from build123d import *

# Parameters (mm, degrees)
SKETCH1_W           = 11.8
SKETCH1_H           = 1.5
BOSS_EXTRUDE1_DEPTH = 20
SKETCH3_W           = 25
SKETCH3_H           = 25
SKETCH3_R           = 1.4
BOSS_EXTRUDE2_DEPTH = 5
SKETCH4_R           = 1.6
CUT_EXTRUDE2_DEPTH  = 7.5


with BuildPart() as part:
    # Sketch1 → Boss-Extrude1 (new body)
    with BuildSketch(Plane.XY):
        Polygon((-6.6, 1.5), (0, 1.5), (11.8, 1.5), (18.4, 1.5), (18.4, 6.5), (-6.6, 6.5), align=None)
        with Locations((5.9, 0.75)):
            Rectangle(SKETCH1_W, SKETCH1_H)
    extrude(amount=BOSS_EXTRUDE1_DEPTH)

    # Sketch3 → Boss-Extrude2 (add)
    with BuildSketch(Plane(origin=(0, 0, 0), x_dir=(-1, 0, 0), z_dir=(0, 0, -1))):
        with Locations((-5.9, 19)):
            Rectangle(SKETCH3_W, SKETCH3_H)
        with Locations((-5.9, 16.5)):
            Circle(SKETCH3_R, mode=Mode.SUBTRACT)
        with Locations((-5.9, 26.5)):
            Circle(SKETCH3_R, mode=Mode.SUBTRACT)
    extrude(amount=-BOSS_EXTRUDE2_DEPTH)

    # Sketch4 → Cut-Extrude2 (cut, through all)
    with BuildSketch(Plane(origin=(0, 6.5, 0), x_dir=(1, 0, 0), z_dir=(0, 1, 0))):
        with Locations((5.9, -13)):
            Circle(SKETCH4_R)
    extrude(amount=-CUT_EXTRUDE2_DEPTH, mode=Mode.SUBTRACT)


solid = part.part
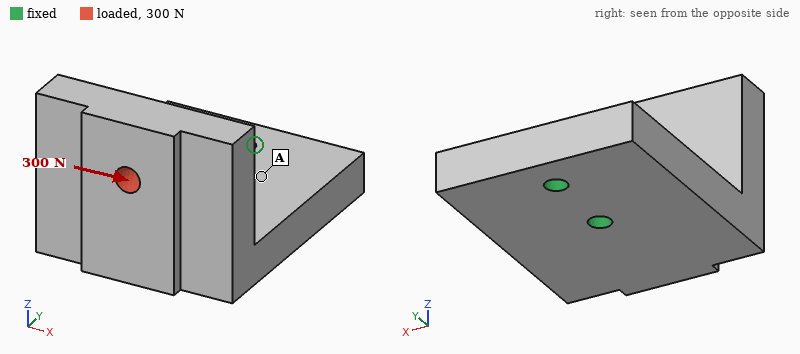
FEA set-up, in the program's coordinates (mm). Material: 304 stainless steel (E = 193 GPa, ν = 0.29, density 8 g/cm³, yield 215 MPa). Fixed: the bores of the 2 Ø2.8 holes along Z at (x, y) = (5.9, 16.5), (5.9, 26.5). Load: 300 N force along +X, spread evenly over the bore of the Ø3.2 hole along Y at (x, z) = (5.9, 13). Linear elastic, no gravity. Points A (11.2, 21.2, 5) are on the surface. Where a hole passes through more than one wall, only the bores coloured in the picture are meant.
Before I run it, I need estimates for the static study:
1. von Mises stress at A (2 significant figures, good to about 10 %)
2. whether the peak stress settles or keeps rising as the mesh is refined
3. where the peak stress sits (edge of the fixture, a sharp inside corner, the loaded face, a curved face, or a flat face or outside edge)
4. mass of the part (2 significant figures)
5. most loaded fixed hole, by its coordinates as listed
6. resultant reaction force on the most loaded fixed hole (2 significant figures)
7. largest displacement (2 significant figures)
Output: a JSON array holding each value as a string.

["7.9 MPa", "keeps rising", "edge of the fixture", "47 g", "(5.9, 16.5)", "600 N", "13 µm"]
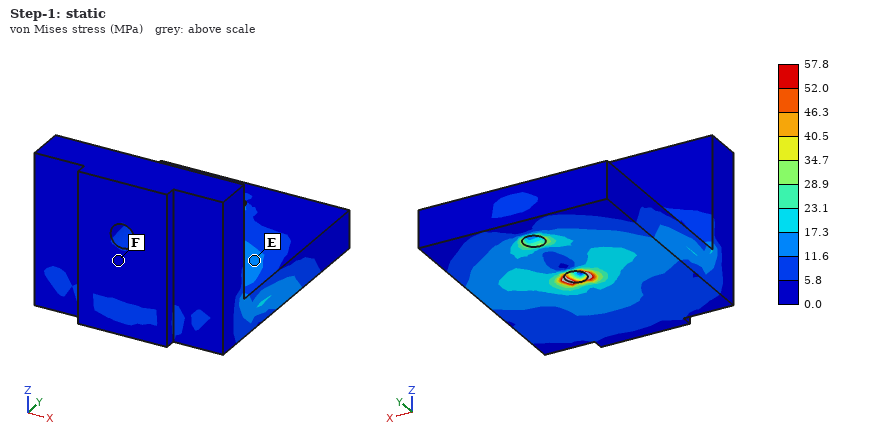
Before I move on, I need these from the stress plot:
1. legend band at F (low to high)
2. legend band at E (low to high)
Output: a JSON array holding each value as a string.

["0.0 to 5.8 MPa", "11.6 to 17.3 MPa"]
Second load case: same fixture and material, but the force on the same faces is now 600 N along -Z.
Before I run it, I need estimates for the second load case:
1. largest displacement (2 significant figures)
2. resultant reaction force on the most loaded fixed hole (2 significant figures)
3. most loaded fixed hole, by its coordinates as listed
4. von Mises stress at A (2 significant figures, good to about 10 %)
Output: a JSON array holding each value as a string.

["29 µm", "900 N", "(5.9, 16.5)", "21 MPa"]
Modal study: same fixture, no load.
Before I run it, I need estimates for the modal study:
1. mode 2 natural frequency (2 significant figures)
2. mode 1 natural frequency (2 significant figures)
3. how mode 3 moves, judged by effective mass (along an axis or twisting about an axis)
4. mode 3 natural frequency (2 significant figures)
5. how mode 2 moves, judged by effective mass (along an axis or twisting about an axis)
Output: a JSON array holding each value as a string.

["6300 Hz", "5000 Hz", "along Z", "14 kHz", "along X"]
